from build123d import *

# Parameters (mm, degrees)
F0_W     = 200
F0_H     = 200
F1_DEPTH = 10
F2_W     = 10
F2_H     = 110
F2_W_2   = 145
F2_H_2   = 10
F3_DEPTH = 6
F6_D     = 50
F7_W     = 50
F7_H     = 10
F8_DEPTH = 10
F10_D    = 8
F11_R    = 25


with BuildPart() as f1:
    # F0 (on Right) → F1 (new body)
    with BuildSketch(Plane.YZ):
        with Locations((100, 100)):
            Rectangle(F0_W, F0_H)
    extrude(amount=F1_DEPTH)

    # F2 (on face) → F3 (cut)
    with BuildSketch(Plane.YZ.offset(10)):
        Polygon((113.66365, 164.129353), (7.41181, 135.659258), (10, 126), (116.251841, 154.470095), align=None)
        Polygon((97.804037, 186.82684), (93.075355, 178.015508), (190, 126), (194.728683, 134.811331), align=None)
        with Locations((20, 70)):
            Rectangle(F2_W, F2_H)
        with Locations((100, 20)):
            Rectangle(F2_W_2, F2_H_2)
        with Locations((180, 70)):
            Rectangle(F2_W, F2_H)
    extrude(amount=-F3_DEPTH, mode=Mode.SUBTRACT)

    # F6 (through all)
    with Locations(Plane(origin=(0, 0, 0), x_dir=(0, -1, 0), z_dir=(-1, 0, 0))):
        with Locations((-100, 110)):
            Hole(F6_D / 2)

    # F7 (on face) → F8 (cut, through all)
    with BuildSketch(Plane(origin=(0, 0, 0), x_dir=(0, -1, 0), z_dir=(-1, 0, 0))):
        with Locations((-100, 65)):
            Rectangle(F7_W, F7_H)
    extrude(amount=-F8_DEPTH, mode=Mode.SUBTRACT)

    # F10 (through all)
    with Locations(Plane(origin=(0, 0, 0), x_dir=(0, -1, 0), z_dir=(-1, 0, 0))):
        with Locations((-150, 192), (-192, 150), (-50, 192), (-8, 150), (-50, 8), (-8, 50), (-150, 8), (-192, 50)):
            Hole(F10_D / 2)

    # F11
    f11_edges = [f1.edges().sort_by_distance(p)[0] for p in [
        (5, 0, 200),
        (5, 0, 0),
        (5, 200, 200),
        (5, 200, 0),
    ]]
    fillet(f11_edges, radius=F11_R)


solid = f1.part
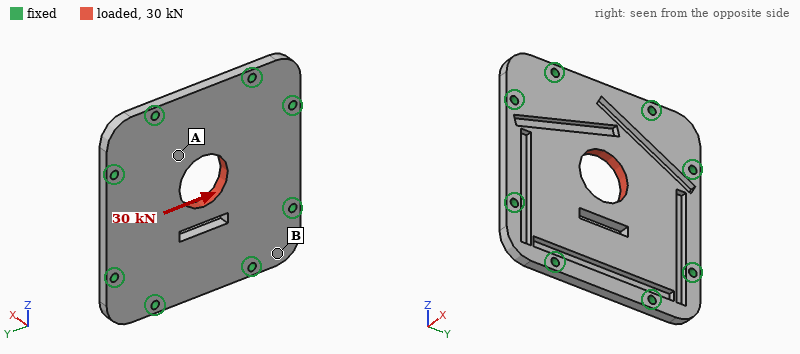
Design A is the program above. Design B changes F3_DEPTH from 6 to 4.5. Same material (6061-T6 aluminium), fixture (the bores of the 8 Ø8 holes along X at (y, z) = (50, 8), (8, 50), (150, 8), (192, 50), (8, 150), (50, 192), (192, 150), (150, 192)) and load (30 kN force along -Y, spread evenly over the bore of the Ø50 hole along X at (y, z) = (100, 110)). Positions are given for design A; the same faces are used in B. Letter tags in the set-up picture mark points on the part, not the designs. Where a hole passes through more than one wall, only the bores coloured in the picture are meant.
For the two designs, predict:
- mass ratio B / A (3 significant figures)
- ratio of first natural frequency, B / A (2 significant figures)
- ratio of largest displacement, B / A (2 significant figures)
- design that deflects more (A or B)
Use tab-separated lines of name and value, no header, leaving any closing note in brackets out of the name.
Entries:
mass ratio B / A	1.03
ratio of first natural frequency, B / A	1.0
ratio of largest displacement, B / A	0.85
design that deflects more	A
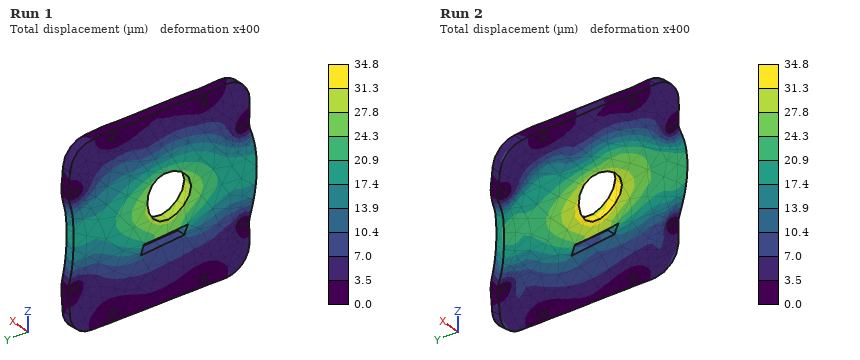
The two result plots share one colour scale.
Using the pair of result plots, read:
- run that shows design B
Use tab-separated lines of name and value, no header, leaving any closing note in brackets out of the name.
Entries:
run that shows design B	Run 1
